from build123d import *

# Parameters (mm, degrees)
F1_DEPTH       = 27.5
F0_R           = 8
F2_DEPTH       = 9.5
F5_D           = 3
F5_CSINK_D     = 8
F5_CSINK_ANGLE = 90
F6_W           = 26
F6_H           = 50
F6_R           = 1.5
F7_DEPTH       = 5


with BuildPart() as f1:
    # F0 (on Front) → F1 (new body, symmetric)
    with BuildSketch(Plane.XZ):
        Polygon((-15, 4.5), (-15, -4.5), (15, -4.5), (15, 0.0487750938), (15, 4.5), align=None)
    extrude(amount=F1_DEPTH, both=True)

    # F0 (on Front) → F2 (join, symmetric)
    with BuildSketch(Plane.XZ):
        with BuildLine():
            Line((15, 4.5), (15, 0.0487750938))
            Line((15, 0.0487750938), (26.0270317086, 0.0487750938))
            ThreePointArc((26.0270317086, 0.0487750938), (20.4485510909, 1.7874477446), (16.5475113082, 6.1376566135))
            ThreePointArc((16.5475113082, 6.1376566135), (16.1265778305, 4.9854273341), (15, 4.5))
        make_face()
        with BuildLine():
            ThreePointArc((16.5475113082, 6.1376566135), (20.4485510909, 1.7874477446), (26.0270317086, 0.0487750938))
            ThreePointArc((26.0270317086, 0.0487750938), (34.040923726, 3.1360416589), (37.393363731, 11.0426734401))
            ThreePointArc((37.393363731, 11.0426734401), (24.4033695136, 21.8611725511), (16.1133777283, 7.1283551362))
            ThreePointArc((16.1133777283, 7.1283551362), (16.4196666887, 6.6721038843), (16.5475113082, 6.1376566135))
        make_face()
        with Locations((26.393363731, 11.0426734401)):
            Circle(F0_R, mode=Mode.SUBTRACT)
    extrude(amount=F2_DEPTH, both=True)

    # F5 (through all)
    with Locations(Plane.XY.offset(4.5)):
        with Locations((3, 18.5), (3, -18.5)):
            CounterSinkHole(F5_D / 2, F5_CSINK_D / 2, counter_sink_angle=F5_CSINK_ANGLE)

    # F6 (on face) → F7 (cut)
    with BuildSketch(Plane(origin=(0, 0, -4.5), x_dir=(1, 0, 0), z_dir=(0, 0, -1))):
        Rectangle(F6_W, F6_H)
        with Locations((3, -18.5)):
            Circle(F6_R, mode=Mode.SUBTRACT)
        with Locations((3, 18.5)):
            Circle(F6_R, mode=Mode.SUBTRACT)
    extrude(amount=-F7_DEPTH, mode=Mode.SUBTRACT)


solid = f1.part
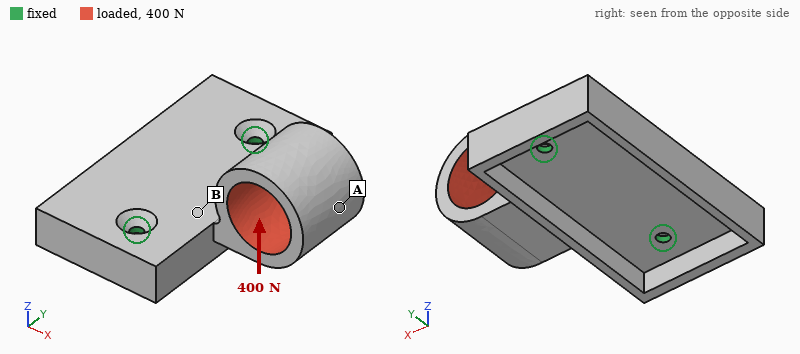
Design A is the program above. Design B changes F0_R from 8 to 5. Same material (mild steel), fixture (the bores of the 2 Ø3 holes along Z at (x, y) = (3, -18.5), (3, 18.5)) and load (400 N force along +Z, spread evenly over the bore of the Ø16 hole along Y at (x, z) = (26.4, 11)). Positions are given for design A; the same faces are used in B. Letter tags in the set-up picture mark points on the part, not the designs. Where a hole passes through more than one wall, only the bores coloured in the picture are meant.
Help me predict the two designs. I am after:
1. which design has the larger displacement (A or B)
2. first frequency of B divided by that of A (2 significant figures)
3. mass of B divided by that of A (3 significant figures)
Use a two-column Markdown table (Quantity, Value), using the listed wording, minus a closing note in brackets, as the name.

| Quantity | Value |
|---|---|
| which design has the larger displacement | A |
| first frequency of B divided by that of A | 0.84 |
| mass of B divided by that of A | 1.19 |
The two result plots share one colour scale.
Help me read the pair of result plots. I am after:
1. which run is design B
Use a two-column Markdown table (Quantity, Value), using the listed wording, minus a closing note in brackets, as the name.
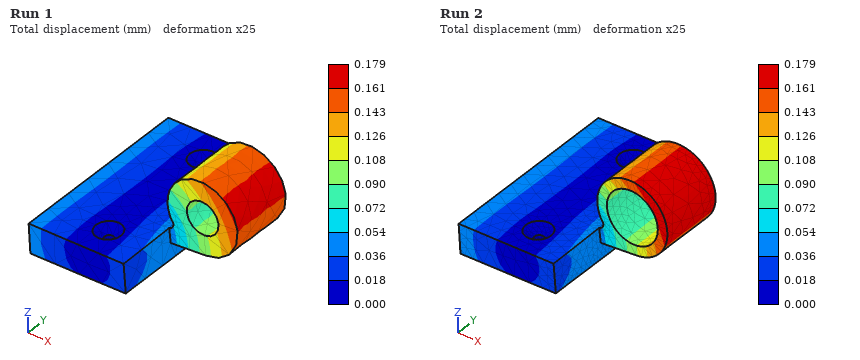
| Quantity | Value |
|---|---|
| which run is design B | Run 1 |
